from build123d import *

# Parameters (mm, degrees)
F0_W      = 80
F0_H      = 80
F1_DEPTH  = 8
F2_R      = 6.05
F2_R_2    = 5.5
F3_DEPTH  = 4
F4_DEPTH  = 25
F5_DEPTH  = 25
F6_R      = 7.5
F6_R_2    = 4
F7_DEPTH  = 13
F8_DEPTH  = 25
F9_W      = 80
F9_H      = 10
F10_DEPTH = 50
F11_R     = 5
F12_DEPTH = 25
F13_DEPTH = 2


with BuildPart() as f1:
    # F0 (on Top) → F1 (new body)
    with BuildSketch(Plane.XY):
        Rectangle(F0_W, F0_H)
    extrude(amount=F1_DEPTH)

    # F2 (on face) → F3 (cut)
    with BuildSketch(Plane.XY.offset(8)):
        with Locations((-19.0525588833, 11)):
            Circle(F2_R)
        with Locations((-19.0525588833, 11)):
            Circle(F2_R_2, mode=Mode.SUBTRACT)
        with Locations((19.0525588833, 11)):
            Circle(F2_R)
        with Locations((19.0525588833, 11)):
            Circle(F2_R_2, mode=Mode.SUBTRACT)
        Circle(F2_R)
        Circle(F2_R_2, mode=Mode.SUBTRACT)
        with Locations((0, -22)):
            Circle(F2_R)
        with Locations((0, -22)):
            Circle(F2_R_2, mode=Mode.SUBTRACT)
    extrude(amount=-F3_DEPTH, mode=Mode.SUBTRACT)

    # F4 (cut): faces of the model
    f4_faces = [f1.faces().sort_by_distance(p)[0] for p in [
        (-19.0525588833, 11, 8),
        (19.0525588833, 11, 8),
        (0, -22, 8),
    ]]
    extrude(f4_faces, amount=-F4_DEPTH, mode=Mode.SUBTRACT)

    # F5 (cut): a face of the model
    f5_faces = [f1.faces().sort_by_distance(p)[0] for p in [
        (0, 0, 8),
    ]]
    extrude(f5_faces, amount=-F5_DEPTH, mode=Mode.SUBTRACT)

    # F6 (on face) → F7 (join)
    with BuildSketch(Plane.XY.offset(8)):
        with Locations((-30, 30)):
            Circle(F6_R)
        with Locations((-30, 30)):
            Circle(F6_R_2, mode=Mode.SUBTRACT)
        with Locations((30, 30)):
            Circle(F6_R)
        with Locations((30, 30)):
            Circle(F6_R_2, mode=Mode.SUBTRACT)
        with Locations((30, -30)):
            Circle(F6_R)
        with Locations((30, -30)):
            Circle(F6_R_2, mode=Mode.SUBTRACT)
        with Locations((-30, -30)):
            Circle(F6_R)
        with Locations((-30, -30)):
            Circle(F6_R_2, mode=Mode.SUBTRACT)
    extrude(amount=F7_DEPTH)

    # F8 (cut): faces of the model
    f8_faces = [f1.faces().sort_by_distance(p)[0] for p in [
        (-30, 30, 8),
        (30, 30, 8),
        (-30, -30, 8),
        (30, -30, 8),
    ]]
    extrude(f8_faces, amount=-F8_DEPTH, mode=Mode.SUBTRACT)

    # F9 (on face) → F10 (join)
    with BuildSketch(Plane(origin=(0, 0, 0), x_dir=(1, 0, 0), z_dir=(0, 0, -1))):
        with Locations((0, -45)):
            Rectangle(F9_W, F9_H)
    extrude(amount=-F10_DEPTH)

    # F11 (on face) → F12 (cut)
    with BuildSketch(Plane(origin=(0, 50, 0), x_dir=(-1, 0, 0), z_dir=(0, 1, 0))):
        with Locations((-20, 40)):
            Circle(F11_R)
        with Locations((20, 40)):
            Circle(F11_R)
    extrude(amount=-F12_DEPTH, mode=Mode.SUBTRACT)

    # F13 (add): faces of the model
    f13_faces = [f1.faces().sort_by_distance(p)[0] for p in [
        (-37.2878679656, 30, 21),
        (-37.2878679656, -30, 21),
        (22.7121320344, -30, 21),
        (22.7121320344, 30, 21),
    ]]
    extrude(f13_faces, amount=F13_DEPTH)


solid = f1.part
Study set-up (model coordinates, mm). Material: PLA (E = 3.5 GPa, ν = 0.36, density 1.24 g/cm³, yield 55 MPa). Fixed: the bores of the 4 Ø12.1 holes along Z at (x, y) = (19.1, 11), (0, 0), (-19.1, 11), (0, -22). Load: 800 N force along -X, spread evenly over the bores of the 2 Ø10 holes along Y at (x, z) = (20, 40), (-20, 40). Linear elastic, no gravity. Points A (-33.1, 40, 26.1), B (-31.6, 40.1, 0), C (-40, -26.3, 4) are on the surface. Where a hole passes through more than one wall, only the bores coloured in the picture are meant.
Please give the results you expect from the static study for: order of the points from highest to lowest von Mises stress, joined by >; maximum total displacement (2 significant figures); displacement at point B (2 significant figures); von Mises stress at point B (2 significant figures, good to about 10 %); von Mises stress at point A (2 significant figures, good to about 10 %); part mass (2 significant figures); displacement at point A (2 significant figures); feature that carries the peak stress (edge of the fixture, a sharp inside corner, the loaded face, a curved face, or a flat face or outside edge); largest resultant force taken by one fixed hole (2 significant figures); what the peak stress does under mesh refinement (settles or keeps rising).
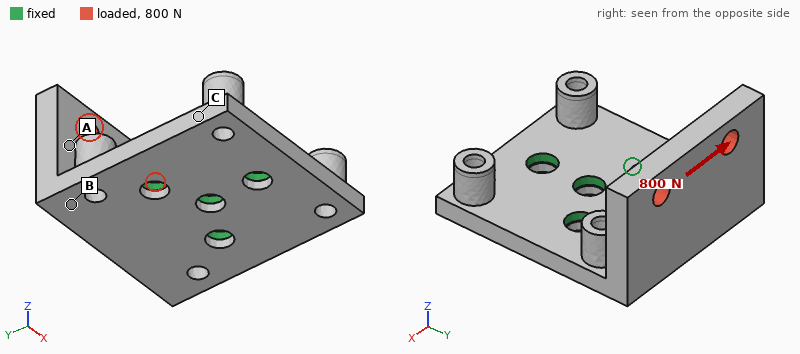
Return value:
B > A > C
1.3 mm
0.55 mm
10 MPa
5.6 MPa
110 g
0.82 mm
edge of the fixture
880 N
keeps rising
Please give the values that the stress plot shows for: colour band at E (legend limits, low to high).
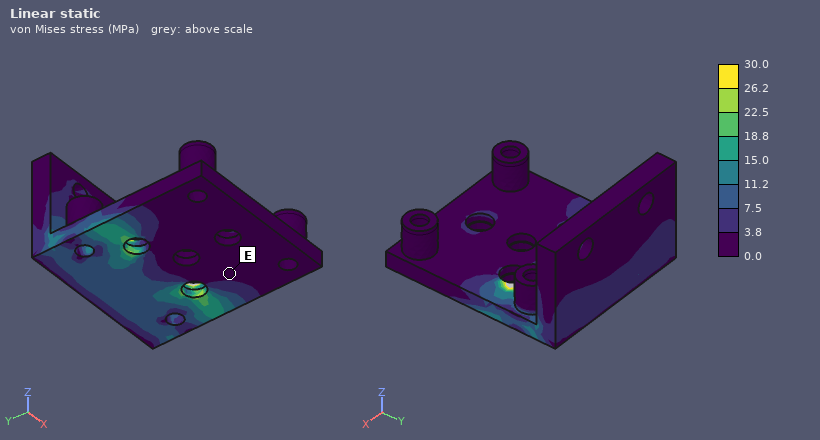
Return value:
0.0 to 3.8 MPa
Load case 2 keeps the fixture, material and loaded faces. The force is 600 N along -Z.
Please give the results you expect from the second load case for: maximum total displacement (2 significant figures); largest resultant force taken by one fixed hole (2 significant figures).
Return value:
1.5 mm
450 N
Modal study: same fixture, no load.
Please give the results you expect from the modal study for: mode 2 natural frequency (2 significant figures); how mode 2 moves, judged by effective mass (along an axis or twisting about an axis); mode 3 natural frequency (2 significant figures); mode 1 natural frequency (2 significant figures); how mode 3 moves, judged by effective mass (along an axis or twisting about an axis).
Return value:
760 Hz
along X
1300 Hz
440 Hz
along Z
